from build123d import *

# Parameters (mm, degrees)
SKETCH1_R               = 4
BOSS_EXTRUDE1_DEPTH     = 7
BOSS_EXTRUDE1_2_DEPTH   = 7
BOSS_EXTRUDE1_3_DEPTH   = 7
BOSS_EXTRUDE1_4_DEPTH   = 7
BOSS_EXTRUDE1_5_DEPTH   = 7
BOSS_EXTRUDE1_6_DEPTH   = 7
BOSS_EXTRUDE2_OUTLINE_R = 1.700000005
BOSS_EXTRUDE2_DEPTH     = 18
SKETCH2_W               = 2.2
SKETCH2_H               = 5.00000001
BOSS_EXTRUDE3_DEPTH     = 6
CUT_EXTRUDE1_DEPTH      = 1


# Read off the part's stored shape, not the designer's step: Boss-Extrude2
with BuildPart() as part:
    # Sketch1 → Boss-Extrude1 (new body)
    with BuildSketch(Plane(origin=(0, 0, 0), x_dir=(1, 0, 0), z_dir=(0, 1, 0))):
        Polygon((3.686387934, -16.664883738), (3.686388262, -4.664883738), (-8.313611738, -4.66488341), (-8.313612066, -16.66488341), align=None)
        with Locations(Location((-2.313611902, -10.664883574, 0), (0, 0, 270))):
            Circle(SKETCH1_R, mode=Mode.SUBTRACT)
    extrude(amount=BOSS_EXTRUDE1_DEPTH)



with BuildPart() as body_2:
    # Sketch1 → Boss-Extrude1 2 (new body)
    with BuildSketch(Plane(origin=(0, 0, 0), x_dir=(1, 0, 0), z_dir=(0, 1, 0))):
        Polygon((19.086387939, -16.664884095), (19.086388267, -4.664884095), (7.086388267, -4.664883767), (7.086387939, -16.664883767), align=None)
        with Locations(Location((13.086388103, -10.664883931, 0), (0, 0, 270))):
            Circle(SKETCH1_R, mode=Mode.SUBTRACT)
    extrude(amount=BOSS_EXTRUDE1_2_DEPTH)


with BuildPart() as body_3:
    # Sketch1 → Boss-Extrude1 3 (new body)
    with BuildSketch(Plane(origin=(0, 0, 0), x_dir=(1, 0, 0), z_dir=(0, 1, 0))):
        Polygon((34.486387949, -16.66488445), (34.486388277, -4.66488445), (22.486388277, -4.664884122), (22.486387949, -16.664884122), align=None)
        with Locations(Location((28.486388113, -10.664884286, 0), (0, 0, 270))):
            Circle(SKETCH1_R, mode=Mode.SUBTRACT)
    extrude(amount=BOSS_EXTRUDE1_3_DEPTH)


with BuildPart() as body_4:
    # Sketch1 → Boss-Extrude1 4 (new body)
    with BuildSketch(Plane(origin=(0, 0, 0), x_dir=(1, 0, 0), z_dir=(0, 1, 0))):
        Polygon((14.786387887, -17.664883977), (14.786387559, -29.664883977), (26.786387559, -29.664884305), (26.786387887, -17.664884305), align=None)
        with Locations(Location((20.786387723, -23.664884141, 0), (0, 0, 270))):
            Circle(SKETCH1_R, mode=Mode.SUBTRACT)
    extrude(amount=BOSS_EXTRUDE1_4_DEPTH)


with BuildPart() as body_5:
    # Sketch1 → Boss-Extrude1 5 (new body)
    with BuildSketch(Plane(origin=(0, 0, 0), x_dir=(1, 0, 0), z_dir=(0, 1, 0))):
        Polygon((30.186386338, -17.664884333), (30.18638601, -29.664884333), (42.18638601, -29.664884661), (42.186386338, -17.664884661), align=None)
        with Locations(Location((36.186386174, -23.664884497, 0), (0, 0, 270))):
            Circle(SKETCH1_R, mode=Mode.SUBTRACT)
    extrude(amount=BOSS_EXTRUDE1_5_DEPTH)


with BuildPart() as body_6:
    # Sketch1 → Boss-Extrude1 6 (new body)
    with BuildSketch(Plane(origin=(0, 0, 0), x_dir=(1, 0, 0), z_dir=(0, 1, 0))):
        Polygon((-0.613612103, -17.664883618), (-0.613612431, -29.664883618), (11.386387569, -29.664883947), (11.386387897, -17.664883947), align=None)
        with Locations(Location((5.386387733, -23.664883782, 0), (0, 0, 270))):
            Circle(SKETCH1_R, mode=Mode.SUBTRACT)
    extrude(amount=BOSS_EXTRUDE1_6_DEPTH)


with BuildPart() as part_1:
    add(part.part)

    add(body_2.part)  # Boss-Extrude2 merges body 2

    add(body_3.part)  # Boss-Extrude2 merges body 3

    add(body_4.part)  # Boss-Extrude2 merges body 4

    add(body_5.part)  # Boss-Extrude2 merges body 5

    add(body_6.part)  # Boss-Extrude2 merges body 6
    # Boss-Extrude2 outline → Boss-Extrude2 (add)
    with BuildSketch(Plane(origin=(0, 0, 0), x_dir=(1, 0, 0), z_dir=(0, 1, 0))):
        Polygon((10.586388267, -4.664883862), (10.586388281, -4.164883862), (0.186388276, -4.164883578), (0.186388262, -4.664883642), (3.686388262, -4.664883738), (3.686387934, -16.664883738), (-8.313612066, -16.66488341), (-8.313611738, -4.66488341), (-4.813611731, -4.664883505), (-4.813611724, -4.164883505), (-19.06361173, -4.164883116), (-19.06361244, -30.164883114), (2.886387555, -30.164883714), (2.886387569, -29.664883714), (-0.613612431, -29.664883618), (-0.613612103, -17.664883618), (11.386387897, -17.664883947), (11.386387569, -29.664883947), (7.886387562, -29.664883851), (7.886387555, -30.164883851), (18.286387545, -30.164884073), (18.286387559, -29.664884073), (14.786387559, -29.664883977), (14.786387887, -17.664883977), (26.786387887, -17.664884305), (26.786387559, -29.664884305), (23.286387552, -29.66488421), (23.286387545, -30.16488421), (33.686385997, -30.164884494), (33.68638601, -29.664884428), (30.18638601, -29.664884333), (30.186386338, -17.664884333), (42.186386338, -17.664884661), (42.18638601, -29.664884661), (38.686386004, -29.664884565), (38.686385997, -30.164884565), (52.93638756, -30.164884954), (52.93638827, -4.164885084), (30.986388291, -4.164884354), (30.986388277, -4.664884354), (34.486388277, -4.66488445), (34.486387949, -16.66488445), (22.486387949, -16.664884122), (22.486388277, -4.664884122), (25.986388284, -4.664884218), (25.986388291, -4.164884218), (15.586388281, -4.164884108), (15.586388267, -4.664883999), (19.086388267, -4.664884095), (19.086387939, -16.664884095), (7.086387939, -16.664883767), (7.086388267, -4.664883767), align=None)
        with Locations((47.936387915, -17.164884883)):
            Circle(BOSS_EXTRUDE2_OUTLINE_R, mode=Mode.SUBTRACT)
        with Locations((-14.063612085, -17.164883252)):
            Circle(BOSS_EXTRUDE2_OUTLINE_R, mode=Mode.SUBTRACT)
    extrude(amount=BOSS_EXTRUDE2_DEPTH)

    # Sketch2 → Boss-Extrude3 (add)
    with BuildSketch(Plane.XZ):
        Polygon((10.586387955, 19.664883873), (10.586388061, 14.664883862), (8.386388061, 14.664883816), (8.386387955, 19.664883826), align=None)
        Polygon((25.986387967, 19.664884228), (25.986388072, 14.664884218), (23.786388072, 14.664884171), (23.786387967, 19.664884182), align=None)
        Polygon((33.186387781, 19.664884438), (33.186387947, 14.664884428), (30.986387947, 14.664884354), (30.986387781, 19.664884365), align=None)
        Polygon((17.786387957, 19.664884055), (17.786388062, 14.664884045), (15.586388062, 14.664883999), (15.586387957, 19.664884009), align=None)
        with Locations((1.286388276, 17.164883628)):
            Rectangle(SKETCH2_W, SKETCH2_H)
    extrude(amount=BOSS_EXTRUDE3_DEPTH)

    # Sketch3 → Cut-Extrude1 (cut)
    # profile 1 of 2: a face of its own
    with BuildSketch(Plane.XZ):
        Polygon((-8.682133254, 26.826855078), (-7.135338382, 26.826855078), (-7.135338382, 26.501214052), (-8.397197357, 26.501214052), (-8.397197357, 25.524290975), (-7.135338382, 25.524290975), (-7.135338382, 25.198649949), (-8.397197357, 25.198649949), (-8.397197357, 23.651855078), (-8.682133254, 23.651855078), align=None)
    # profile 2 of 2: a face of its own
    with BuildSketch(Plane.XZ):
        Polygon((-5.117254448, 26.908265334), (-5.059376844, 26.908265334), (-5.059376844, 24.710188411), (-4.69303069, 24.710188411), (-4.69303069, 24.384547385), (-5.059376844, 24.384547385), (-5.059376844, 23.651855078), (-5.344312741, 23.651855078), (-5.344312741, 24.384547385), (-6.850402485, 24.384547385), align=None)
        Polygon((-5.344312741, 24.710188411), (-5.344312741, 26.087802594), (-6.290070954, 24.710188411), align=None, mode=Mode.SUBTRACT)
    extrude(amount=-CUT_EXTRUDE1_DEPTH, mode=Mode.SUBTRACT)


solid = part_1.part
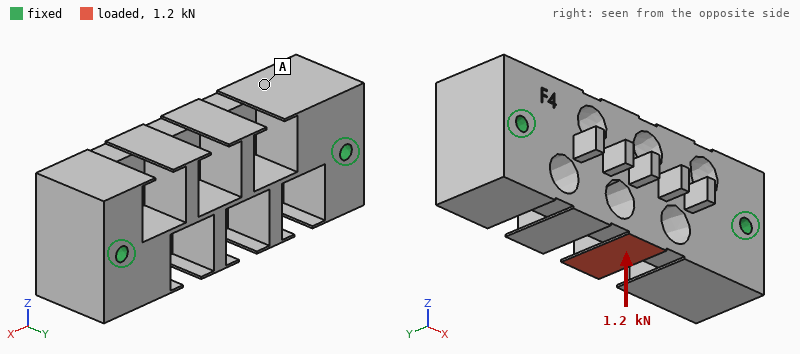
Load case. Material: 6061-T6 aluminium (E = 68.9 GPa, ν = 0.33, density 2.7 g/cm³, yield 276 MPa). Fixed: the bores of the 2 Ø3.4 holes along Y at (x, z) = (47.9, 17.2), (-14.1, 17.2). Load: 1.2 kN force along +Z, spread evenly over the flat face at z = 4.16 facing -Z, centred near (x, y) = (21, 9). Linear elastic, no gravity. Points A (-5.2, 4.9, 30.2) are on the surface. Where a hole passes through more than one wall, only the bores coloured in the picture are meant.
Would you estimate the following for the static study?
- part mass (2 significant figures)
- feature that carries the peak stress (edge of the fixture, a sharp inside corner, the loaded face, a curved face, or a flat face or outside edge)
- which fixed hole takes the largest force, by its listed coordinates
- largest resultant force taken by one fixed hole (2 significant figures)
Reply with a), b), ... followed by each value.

a) 59 g
b) the loaded face
c) (47.9, 17.2)
d) 690 N
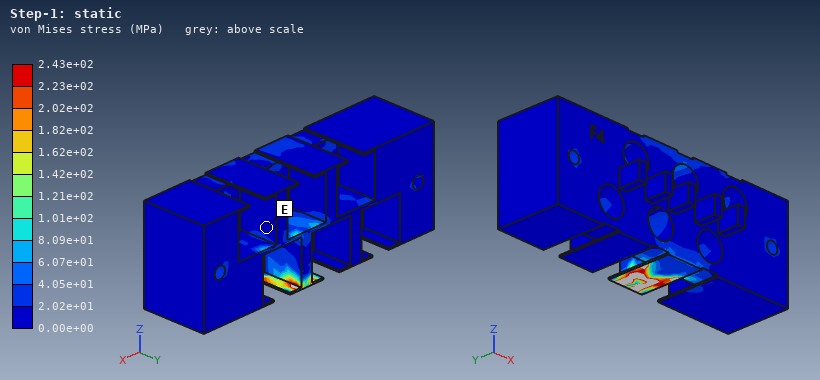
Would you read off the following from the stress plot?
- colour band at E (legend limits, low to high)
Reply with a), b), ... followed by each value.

a) 0.00e+00 to 2.02e+01 MPa
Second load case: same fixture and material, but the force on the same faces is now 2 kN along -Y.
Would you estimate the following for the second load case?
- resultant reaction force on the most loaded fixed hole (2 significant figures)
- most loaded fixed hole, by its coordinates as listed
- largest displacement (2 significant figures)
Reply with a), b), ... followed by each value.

a) 1.3 kN
b) (47.9, 17.2)
c) 0.13 mm
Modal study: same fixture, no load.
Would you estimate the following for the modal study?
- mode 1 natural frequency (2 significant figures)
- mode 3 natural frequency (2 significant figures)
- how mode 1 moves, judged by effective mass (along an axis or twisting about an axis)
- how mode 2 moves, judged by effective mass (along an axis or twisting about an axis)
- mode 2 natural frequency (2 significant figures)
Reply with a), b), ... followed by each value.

a) 10 kHz
b) 13 kHz
c) along Z
d) along Y
e) 11 kHz
